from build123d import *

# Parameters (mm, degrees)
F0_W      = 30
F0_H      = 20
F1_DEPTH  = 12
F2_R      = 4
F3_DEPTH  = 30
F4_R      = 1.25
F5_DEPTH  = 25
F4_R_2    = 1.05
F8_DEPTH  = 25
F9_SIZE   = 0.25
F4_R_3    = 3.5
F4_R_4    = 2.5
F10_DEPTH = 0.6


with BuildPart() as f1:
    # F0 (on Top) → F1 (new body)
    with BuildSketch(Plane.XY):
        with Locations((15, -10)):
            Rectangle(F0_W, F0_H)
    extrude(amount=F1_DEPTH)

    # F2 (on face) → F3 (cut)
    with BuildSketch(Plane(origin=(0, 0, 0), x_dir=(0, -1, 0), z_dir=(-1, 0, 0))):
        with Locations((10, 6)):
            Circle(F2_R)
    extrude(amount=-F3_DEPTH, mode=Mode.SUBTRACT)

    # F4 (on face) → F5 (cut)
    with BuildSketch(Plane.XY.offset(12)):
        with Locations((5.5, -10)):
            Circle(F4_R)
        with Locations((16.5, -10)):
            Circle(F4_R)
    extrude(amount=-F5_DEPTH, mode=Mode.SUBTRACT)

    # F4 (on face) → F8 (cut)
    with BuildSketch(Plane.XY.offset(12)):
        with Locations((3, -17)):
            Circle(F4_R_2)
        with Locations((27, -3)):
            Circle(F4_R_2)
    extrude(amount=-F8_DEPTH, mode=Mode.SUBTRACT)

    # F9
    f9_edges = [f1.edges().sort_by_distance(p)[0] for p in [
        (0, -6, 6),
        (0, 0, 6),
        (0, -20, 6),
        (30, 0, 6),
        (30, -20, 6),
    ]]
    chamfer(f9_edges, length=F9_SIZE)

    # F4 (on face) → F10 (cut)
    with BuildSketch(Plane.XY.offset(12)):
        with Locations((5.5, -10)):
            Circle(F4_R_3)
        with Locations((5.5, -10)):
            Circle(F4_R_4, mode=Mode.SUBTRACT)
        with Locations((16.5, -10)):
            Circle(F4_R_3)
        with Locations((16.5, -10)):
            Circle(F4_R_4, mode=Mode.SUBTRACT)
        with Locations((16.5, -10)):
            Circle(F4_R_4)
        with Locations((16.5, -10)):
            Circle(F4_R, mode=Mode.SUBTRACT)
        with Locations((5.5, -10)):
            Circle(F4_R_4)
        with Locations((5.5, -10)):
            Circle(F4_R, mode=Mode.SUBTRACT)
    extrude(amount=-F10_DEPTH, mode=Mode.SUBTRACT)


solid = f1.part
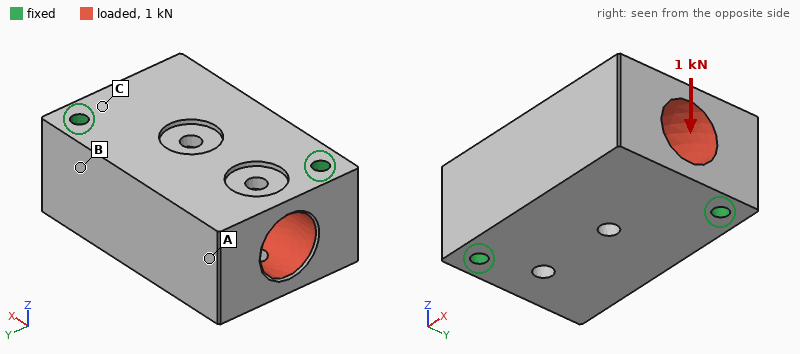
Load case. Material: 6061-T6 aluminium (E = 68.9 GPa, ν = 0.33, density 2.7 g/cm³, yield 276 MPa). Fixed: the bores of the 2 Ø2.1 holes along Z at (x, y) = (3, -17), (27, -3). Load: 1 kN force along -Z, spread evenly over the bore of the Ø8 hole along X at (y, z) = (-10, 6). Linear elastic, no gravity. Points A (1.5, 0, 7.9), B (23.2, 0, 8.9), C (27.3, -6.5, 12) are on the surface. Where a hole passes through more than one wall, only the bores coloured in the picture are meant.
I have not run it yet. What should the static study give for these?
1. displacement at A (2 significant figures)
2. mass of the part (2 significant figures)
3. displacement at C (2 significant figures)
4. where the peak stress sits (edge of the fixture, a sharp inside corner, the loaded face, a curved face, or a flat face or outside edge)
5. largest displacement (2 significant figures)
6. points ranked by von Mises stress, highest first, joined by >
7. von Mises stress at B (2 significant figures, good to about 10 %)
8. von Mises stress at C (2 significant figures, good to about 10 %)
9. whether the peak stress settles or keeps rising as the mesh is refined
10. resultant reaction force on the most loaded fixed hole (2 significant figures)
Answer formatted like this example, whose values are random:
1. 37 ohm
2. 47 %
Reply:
1. 4.5 µm
2. 15 g
3. 0.99 µm
4. edge of the fixture
5. 4.8 µm
6. C > B > A
7. 5.5 MPa
8. 12 MPa
9. keeps rising
10. 510 N
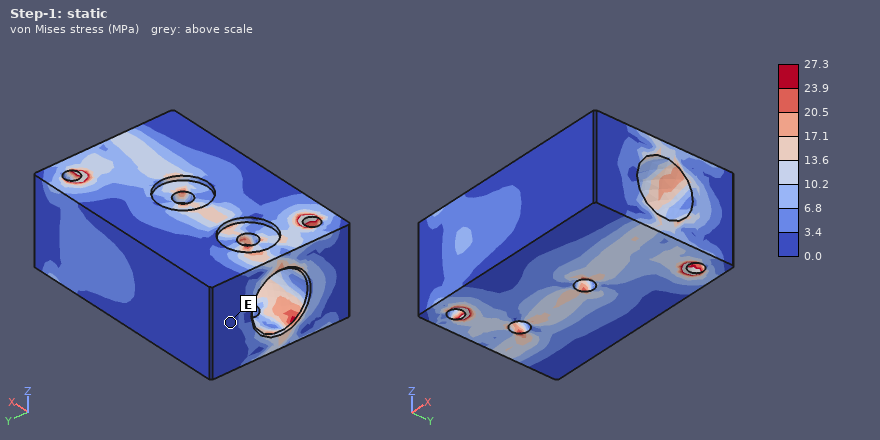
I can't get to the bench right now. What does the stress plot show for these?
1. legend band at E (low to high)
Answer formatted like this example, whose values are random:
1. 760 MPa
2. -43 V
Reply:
1. 0.0 to 3.4 MPa
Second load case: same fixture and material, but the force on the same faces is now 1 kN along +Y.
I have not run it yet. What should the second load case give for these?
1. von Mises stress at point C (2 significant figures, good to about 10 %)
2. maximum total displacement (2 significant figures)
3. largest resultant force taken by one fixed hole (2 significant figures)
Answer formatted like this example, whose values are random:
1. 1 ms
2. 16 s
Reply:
1. 12 MPa
2. 1.9 µm
3. 520 N
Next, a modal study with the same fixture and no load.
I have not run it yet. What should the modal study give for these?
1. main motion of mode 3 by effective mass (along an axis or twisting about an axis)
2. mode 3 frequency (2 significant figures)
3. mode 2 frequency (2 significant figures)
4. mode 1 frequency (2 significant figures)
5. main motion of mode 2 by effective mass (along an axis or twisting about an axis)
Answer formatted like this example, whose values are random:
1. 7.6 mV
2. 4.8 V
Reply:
1. along Y
2. 32 kHz
3. 22 kHz
4. 18 kHz
5. along Z
